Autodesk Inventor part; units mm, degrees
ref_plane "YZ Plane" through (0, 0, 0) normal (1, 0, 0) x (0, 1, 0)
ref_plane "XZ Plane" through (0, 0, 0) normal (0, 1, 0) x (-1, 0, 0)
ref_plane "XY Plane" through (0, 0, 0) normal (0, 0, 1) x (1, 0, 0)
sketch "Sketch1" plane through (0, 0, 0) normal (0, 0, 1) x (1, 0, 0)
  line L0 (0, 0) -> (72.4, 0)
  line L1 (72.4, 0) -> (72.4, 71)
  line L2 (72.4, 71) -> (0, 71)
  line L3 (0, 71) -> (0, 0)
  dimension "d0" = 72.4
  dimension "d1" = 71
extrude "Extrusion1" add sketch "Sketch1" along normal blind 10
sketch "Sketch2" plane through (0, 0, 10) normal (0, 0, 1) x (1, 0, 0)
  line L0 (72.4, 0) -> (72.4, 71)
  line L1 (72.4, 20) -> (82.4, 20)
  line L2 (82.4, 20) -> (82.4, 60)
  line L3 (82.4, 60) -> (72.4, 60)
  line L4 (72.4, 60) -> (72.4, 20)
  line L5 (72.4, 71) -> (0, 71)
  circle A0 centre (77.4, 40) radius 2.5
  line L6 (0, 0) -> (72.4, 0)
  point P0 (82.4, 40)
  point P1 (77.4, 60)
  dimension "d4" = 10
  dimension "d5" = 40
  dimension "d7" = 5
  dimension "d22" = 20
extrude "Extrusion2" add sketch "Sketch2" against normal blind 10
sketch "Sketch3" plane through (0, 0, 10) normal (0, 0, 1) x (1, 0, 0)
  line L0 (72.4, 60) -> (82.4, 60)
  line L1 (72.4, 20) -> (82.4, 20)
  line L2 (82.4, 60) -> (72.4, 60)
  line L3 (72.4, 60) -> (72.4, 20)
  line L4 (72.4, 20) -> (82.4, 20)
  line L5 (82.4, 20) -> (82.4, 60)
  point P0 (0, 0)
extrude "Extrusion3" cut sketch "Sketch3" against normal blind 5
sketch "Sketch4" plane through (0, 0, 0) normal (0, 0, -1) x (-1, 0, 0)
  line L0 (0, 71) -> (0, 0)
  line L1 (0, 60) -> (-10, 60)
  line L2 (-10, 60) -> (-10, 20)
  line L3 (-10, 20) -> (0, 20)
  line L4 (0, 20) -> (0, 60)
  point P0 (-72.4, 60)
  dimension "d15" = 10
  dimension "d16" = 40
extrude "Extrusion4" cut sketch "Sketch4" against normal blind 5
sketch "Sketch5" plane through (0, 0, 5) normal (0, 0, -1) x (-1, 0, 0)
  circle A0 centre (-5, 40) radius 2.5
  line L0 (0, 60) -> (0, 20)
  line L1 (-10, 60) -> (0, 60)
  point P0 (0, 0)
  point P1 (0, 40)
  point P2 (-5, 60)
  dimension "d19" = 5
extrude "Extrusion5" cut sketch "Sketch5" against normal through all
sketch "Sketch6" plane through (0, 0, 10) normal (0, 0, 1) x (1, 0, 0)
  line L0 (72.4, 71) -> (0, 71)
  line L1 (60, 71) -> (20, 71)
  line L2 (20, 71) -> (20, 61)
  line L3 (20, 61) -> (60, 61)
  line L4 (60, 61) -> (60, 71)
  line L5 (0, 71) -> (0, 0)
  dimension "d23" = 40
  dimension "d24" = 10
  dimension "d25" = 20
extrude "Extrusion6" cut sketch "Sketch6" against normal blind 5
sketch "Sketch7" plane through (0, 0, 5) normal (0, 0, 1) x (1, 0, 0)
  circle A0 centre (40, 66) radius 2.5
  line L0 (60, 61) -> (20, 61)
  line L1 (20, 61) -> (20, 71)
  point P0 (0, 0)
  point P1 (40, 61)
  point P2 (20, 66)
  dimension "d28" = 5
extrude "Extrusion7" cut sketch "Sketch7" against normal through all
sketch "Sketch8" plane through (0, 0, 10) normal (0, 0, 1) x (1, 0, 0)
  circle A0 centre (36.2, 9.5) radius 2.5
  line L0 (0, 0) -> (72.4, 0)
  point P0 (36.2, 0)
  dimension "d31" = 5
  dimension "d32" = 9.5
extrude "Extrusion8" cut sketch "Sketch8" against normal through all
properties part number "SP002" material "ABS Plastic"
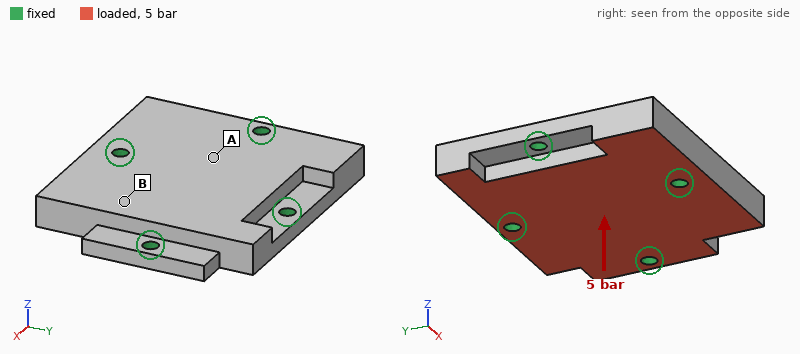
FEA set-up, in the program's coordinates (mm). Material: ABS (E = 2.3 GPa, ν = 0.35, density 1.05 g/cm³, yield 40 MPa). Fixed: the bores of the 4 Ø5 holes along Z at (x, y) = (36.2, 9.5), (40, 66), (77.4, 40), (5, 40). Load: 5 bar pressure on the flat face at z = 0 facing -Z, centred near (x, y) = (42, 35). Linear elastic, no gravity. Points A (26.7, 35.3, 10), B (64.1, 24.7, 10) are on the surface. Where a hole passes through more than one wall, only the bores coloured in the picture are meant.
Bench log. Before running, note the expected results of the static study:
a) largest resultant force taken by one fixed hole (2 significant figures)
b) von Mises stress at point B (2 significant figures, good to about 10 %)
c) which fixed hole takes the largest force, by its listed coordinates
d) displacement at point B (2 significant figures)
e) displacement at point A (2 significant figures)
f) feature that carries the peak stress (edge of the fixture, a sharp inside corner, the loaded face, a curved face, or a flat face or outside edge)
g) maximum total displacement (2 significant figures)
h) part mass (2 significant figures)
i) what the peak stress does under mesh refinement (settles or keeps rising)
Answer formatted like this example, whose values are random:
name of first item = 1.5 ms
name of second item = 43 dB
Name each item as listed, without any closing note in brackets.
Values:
largest resultant force taken by one fixed hole = 920 N
von Mises stress at point B = 6.2 MPa
which fixed hole takes the largest force, by its listed coordinates = (36.2, 9.5)
displacement at point B = 0.15 mm
displacement at point A = 0.10 mm
feature that carries the peak stress = edge of the fixture
maximum total displacement = 0.34 mm
part mass = 51 g
what the peak stress does under mesh refinement = keeps rising
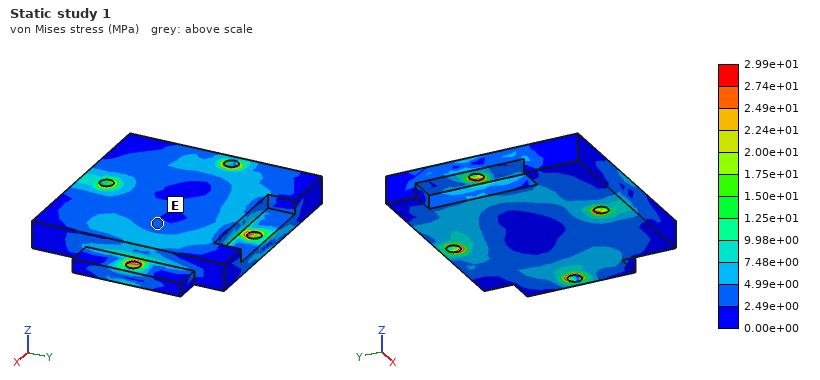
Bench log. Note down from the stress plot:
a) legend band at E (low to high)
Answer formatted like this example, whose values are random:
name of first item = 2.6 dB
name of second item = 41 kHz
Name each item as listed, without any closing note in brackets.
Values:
legend band at E = 2.49e+00 to 4.99e+00 MPa
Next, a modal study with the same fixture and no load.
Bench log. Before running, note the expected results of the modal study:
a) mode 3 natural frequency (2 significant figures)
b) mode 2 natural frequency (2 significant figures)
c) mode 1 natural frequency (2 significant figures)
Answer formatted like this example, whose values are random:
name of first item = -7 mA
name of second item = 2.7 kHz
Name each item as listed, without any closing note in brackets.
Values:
mode 3 natural frequency = 2600 Hz
mode 2 natural frequency = 2400 Hz
mode 1 natural frequency = 2200 Hz
